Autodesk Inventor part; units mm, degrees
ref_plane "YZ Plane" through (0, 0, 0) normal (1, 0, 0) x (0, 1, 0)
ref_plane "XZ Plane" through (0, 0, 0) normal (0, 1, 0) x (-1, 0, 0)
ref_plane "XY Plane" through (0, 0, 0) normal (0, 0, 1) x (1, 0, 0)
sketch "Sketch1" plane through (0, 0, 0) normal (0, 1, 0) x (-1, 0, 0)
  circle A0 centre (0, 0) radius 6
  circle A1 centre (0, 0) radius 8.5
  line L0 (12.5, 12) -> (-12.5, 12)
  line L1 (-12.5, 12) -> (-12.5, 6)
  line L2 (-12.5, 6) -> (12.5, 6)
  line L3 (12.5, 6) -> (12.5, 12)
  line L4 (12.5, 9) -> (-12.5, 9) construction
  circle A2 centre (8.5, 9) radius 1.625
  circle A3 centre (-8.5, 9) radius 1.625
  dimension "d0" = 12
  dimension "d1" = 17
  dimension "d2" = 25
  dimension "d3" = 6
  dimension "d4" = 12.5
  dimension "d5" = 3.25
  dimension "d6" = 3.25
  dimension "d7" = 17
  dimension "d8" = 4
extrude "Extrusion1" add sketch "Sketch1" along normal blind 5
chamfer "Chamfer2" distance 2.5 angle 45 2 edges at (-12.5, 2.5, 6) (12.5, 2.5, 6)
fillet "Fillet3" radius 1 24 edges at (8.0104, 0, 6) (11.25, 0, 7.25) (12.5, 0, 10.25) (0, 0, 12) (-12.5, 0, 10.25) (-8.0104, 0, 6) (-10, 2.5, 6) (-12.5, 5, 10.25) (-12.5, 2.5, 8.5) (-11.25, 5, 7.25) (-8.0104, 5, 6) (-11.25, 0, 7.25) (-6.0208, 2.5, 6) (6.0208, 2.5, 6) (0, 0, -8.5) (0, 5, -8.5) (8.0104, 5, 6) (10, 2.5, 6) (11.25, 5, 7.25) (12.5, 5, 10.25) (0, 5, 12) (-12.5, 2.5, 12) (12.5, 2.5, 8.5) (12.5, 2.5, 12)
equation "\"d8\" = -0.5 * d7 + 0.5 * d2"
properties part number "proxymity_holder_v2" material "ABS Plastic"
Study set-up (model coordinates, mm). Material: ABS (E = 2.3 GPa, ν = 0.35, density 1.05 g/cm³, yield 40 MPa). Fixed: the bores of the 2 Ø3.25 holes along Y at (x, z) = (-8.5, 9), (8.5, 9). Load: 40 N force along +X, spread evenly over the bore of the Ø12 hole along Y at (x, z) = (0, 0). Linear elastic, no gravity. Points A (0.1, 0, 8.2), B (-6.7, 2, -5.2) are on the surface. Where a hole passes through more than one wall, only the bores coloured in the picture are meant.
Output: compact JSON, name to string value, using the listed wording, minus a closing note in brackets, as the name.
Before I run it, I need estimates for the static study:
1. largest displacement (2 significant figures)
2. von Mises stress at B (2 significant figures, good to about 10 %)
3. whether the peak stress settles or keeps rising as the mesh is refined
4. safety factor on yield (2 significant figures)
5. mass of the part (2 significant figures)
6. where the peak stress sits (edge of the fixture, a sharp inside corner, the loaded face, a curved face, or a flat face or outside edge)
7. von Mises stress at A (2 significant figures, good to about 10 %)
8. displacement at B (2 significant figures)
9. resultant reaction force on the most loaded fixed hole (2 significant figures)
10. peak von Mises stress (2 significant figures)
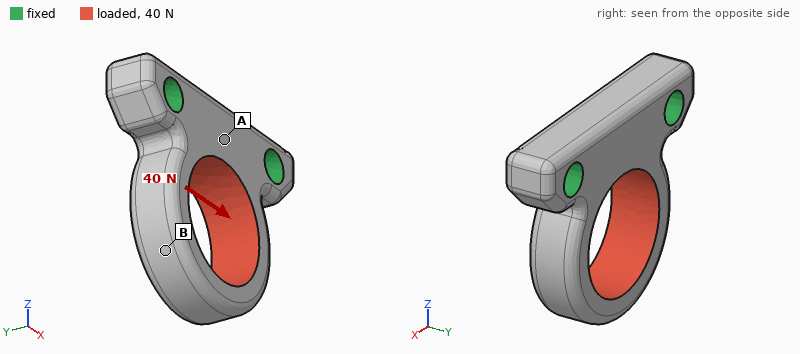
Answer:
{"largest displacement": "0.12 mm", "von Mises stress at B": "4.6 MPa", "whether the peak stress settles or keeps rising as the mesh is refined": "settles", "safety factor on yield": "2.5", "mass of the part": "1.1 g", "where the peak stress sits": "a curved face", "von Mises stress at A": "1.4 MPa", "displacement at B": "0.11 mm", "resultant reaction force on the most loaded fixed hole": "29 N", "peak von Mises stress": "16 MPa"}
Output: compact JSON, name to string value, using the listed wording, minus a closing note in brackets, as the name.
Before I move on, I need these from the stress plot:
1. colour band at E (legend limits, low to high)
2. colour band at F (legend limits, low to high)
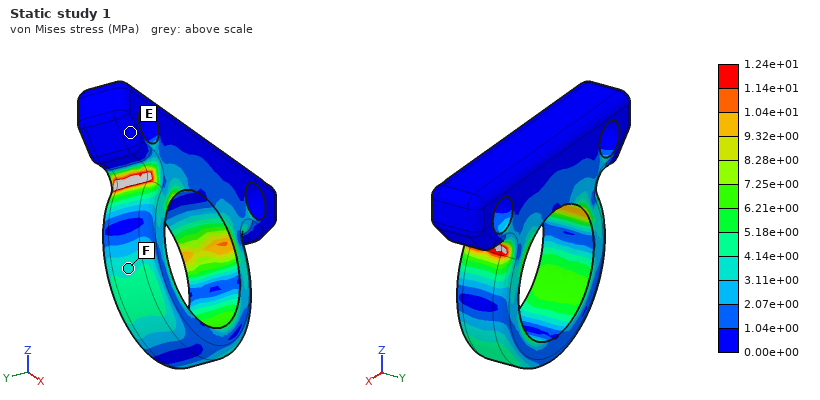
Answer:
{"colour band at E": "0.00e+00 to 1.04e+00 MPa", "colour band at F": "3.11e+00 to 4.14e+00 MPa"}
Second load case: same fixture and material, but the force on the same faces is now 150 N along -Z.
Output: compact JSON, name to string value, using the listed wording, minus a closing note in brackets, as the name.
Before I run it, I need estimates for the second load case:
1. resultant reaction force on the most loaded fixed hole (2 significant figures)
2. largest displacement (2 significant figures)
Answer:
{"resultant reaction force on the most loaded fixed hole": "77 N", "largest displacement": "72 µm"}
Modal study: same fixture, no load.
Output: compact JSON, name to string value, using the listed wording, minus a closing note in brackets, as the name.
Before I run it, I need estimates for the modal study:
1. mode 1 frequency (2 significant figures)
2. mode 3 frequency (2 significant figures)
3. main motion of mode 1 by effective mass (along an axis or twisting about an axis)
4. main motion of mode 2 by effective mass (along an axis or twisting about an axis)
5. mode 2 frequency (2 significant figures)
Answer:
{"mode 1 frequency": "3300 Hz", "mode 3 frequency": "7600 Hz", "main motion of mode 1 by effective mass": "along Y", "main motion of mode 2 by effective mass": "along X", "mode 2 frequency": "4200 Hz"}
